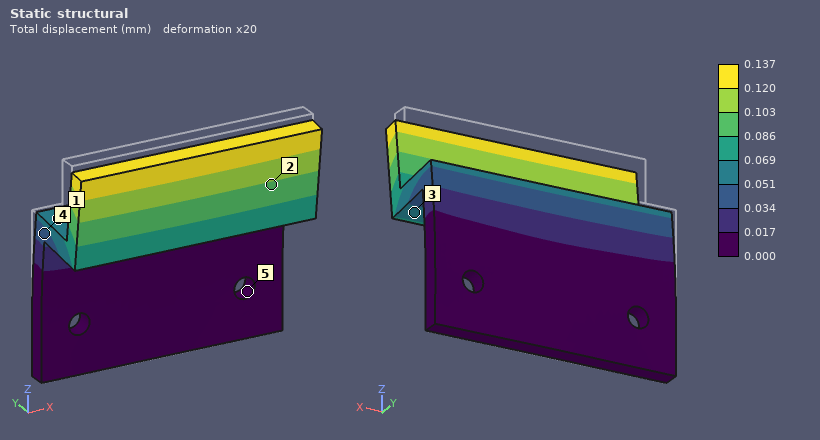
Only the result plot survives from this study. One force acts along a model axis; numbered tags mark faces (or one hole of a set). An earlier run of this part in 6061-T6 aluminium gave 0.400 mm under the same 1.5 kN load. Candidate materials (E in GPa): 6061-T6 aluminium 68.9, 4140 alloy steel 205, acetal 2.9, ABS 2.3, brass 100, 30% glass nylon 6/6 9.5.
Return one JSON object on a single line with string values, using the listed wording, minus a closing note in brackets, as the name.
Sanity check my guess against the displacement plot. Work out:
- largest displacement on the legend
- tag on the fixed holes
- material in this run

{"largest displacement on the legend": "0.137 mm", "tag on the fixed holes": "5", "material in this run": "4140 alloy steel"}
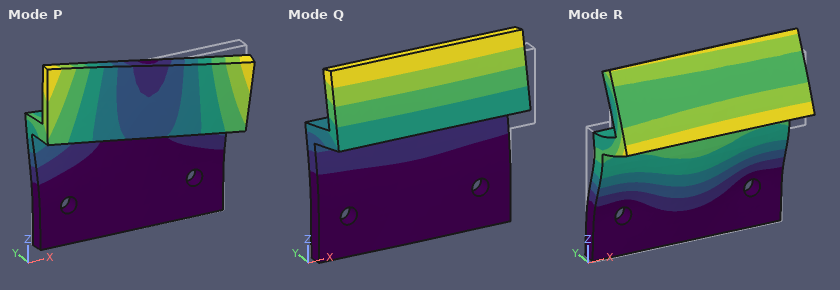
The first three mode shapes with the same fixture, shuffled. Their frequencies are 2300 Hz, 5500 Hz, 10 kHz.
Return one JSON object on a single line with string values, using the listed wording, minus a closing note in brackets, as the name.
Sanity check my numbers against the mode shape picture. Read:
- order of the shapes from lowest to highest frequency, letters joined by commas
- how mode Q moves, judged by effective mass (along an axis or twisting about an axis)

{"order of the shapes from lowest to highest frequency, letters joined by commas": "Q, P, R", "how mode Q moves, judged by effective mass": "along Y"}
